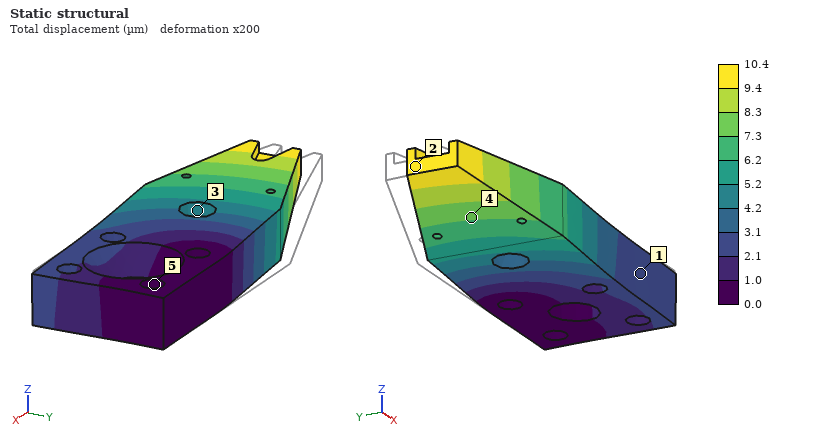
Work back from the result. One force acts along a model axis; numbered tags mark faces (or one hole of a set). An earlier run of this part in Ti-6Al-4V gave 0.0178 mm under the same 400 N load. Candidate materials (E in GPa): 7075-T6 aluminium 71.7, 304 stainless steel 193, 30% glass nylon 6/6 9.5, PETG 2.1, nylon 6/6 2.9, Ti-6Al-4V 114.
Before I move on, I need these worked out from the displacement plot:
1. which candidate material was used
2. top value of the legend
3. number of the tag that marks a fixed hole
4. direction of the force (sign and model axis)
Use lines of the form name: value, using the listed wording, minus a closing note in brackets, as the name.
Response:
which candidate material was used: 304 stainless steel
top value of the legend: 10.4 µm
number of the tag that marks a fixed hole: 5
direction of the force: -Y
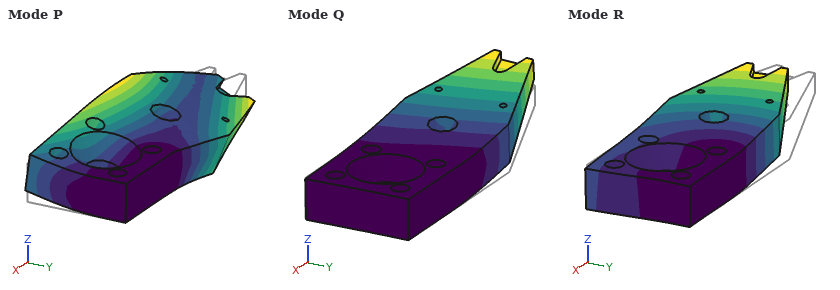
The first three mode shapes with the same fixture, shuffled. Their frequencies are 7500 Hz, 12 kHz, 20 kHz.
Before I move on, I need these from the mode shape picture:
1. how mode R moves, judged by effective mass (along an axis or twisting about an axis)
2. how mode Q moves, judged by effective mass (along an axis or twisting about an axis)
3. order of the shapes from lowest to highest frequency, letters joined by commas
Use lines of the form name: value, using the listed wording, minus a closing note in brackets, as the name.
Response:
how mode R moves, judged by effective mass: along Y
how mode Q moves, judged by effective mass: along Z
order of the shapes from lowest to highest frequency, letters joined by commas: Q, R, P
